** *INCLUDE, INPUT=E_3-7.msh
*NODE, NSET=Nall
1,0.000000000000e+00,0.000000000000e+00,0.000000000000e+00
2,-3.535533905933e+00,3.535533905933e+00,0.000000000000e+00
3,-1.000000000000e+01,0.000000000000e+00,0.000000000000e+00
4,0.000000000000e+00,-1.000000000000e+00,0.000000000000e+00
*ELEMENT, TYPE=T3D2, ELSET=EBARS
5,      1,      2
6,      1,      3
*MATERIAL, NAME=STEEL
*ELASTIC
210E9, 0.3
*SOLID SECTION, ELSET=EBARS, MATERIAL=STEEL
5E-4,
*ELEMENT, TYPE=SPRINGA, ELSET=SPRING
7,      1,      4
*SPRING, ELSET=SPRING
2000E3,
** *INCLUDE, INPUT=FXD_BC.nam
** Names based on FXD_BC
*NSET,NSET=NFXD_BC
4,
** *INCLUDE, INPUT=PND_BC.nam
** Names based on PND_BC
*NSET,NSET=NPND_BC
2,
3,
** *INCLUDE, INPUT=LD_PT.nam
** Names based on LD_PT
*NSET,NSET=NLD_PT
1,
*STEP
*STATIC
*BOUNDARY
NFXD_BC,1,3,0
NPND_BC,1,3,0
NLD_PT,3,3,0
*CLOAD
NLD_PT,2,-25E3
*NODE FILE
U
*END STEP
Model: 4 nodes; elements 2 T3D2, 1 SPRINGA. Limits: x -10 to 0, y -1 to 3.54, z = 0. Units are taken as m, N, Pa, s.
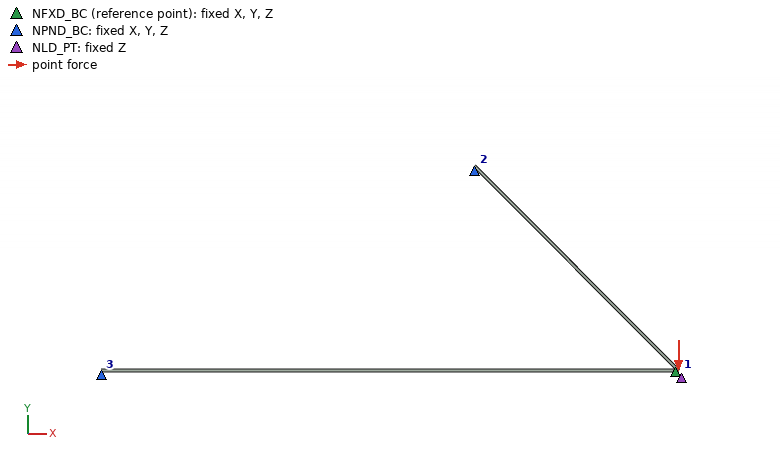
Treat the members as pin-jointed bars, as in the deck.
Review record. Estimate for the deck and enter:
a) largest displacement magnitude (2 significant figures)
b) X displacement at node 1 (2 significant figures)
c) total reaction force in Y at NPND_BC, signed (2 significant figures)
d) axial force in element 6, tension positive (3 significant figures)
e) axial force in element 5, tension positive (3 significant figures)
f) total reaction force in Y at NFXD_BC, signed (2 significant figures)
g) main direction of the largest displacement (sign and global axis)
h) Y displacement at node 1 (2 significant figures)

0.0039 m
-0.0017 m
18000 N
-18100 N
25600 N
6900 N
-Y
-0.0034 m
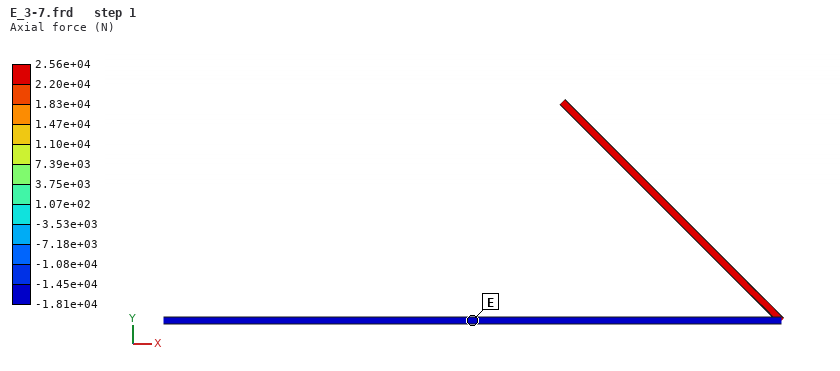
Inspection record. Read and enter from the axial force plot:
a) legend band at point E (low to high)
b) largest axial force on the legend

-1.81e+04 to -1.45e+04 N
2.56e+04 N
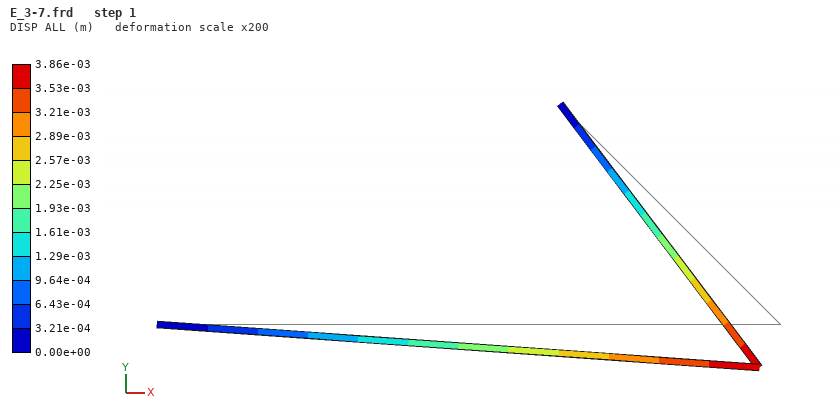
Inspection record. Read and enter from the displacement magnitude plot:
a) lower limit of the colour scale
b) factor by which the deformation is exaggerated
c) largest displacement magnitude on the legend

0.00e+00 m
200
3.86e-03 m
